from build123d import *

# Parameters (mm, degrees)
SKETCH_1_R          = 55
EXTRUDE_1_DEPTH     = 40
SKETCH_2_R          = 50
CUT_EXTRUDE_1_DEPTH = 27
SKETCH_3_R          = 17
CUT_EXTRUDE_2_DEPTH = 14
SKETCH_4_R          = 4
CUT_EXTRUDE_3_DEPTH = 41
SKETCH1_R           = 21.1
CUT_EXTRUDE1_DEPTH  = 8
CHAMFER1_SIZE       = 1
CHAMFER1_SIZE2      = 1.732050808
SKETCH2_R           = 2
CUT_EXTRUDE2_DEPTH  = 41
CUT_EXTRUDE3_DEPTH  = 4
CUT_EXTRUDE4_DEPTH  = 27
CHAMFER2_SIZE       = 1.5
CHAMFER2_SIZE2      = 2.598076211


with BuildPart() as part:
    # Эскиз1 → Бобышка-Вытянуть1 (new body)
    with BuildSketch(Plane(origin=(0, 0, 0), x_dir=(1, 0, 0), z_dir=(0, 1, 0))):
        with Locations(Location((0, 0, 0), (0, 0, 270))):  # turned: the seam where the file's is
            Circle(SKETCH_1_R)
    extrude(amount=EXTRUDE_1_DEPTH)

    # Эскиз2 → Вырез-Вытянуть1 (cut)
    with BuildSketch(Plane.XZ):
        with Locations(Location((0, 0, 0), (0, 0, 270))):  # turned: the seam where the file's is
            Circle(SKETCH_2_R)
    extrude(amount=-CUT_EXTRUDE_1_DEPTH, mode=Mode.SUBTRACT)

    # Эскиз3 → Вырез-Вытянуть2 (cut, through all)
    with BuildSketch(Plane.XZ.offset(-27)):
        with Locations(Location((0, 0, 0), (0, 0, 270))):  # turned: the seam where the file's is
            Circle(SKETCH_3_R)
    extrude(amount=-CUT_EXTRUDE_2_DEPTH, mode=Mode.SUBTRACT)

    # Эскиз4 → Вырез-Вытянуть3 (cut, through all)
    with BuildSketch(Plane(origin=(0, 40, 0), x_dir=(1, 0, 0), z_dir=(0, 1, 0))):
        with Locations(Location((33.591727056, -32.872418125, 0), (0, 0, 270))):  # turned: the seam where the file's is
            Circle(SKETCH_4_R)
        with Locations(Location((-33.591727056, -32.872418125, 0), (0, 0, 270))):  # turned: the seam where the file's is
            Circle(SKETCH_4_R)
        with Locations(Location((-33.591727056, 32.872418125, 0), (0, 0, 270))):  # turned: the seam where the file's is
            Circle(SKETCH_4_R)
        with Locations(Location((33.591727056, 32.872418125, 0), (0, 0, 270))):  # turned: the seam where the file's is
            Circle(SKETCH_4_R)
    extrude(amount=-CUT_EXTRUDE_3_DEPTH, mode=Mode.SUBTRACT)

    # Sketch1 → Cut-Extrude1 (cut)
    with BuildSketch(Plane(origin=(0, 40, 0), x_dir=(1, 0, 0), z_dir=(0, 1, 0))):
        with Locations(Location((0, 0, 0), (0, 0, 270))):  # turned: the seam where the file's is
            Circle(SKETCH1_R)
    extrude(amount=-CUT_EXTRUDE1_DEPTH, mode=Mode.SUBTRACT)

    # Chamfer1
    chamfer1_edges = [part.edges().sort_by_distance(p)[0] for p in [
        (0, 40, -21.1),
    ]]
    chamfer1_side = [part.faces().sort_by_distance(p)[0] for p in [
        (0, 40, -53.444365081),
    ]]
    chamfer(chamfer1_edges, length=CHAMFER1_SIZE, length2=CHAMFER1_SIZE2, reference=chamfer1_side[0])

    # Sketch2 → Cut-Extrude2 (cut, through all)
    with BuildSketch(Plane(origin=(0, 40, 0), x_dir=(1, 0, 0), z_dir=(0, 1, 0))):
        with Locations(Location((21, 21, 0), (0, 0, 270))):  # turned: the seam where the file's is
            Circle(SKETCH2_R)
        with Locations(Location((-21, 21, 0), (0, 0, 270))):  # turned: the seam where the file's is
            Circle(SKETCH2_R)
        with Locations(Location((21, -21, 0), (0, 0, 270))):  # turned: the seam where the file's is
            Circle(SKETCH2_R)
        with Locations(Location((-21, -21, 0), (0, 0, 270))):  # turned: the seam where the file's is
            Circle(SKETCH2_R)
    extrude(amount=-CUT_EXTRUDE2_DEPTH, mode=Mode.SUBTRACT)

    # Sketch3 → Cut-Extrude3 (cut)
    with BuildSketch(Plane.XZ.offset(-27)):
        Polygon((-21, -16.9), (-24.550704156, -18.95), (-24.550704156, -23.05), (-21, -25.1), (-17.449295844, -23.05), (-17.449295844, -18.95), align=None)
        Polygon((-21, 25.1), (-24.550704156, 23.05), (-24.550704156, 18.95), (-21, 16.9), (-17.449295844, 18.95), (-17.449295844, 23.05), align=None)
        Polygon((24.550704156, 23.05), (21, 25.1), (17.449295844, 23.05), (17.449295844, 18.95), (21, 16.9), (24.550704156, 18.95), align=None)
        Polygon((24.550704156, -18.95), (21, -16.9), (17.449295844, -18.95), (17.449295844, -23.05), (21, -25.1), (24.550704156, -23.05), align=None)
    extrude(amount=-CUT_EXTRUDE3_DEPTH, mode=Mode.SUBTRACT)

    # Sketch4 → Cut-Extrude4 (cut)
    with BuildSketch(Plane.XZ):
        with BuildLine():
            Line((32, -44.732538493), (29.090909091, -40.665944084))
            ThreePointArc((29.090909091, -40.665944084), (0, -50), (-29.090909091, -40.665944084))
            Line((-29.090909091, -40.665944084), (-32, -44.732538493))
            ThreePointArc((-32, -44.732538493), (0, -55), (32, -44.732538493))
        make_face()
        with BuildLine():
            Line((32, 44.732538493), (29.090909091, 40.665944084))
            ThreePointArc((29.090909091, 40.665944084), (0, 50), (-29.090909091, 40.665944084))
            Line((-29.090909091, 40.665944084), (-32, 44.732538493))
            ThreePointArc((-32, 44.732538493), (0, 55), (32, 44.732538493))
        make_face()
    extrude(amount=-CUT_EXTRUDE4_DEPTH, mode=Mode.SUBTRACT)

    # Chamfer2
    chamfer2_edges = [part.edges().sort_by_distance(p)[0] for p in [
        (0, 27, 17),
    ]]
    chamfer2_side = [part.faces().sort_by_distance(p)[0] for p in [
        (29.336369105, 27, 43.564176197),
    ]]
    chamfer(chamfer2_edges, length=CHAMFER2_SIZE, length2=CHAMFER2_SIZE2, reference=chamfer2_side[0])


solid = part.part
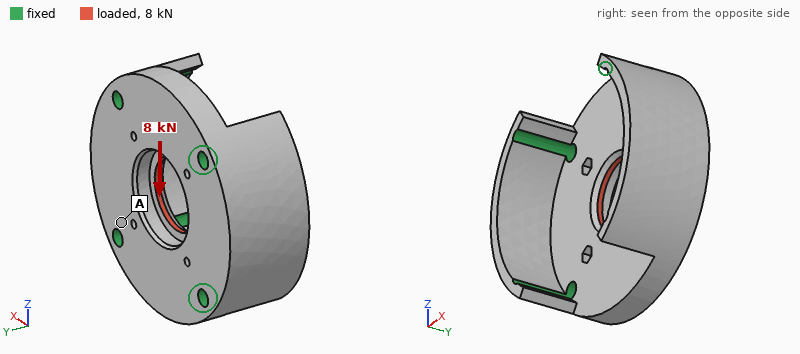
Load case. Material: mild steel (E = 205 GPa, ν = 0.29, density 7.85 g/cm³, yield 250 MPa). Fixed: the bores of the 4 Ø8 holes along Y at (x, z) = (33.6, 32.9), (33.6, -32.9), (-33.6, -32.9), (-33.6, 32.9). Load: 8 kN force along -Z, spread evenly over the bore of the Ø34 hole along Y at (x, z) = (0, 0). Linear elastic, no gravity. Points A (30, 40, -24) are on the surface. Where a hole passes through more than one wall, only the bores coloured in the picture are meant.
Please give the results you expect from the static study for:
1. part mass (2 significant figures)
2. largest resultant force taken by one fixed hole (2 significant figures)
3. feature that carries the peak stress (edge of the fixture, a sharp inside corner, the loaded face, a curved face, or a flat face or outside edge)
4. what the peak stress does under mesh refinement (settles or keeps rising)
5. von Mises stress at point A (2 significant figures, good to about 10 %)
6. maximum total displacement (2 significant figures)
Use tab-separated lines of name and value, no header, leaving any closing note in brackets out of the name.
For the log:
part mass	1.0 kg
largest resultant force taken by one fixed hole	2.0 kN
feature that carries the peak stress	a sharp inside corner
what the peak stress does under mesh refinement	keeps rising
von Mises stress at point A	7.2 MPa
maximum total displacement	2.5 µm
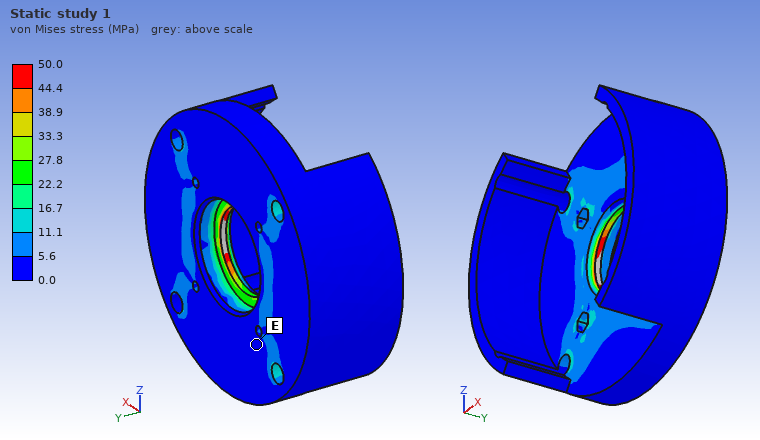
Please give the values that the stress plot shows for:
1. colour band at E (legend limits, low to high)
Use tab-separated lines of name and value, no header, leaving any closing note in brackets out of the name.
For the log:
colour band at E	0.0 to 5.6 MPa
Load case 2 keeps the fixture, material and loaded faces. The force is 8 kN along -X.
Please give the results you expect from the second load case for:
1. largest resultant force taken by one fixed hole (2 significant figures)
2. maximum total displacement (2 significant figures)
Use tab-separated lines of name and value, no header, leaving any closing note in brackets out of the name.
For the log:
largest resultant force taken by one fixed hole	2.0 kN
maximum total displacement	2.4 µm
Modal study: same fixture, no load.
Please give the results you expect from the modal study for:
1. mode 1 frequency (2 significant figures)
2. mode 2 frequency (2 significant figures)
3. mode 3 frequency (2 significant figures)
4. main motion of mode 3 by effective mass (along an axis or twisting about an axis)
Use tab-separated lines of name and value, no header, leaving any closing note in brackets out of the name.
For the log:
mode 1 frequency	11 kHz
mode 2 frequency	11 kHz
mode 3 frequency	12 kHz
main motion of mode 3 by effective mass	along Y
